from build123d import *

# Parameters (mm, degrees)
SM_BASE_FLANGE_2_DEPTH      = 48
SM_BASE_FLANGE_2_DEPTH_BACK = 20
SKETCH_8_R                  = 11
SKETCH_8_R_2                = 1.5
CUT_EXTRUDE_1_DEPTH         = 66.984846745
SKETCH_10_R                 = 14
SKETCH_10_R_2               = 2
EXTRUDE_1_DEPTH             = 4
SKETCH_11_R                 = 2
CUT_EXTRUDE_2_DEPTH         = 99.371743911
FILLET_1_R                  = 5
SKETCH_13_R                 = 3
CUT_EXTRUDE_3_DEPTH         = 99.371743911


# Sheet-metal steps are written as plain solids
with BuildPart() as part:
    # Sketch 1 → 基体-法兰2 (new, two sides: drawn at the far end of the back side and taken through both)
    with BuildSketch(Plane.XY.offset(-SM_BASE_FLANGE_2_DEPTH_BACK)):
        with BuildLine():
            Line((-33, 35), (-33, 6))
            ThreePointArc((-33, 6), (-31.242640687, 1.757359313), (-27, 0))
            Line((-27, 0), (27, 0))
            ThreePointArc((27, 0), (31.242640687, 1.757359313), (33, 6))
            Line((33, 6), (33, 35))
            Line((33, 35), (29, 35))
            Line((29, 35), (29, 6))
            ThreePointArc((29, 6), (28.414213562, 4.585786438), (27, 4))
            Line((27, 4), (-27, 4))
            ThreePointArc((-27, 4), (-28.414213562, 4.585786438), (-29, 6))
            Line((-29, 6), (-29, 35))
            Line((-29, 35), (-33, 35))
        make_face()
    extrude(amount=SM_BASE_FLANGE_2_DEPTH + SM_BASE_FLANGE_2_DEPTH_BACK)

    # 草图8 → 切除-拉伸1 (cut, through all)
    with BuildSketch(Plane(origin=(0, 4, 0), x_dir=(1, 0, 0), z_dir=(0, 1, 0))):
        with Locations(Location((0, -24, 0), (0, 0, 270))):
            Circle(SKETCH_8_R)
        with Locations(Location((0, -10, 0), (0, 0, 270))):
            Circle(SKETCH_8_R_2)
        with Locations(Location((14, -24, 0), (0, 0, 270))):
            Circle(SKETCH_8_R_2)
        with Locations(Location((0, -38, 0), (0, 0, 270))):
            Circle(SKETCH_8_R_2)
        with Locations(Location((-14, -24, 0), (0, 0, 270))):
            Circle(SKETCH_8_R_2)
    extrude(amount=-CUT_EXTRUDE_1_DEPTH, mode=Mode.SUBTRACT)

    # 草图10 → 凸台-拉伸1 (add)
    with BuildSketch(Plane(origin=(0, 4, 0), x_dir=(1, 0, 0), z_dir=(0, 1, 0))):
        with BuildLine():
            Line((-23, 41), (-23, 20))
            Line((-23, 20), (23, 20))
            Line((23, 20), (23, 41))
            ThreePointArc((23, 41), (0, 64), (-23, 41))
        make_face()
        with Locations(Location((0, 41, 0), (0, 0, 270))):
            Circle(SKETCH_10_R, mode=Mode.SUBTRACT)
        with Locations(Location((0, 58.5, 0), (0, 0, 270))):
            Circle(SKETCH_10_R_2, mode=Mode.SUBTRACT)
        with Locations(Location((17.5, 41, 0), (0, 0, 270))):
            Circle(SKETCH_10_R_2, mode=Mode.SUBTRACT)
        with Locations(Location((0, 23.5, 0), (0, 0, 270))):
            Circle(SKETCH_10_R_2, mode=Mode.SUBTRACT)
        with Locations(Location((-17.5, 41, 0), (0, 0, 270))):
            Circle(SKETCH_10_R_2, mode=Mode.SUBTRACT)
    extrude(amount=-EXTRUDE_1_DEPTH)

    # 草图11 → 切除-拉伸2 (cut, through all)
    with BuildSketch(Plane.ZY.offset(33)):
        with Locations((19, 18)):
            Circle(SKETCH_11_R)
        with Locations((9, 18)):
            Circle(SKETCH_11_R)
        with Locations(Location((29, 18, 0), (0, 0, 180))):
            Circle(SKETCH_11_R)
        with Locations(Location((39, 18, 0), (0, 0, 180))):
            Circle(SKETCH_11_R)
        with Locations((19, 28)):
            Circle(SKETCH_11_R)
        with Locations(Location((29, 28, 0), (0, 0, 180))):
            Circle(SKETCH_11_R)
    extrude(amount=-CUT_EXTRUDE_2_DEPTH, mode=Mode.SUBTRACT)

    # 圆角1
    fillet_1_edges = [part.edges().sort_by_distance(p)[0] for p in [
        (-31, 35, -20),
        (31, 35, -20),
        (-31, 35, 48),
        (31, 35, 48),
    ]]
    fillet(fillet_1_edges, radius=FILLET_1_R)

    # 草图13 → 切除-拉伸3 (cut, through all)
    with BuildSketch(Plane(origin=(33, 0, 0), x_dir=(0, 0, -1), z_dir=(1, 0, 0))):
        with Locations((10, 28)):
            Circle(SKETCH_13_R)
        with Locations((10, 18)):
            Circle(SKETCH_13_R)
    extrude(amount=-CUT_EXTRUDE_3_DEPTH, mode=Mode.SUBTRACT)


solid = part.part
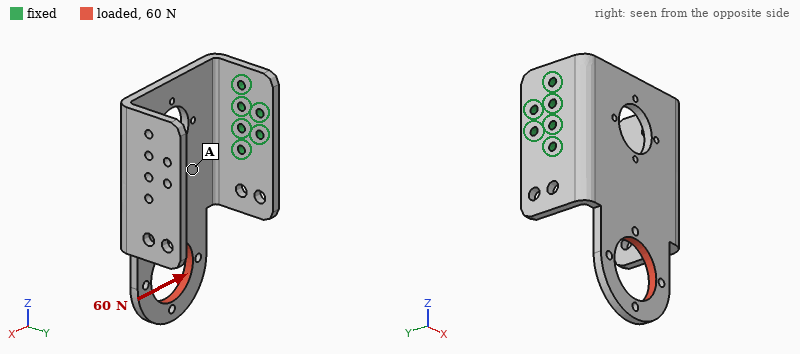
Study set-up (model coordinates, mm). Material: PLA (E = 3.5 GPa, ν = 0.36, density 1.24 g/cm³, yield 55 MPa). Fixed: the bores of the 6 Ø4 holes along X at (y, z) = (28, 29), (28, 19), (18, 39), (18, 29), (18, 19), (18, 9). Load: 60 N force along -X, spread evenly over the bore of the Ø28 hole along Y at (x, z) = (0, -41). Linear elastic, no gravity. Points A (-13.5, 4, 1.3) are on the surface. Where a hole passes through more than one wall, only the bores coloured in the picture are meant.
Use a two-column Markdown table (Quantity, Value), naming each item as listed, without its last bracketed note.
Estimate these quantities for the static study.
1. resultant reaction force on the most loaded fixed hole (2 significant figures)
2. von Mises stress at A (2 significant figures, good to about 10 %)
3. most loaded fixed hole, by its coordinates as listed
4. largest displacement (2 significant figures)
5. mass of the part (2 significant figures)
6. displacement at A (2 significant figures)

| Quantity | Value |
|---|---|
| resultant reaction force on the most loaded fixed hole | 150 N |
| von Mises stress at A | 2.3 MPa |
| most loaded fixed hole, by its coordinates as listed | (18, 9) |
| largest displacement | 1.5 mm |
| mass of the part | 44 g |
| displacement at A | 0.42 mm |
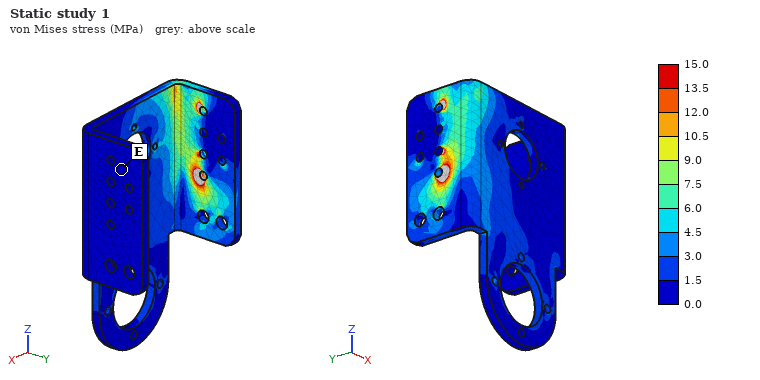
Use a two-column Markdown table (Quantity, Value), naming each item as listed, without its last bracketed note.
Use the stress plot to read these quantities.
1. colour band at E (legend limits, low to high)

| Quantity | Value |
|---|---|
| colour band at E | 0.0 to 1.5 MPa |
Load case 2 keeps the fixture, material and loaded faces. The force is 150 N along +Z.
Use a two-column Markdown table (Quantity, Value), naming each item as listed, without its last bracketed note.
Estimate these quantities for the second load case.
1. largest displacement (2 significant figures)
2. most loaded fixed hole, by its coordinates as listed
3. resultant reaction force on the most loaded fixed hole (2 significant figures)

| Quantity | Value |
|---|---|
| largest displacement | 1.5 mm |
| most loaded fixed hole, by its coordinates as listed | (18, 9) |
| resultant reaction force on the most loaded fixed hole | 170 N |
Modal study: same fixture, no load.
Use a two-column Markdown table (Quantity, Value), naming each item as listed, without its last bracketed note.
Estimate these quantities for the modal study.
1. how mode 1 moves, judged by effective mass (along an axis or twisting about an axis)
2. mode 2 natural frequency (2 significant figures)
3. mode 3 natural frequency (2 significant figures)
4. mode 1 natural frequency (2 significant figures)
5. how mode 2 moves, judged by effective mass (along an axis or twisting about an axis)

| Quantity | Value |
|---|---|
| how mode 1 moves, judged by effective mass | along Y |
| mode 2 natural frequency | 210 Hz |
| mode 3 natural frequency | 350 Hz |
| mode 1 natural frequency | 110 Hz |
| how mode 2 moves, judged by effective mass | along Z |
